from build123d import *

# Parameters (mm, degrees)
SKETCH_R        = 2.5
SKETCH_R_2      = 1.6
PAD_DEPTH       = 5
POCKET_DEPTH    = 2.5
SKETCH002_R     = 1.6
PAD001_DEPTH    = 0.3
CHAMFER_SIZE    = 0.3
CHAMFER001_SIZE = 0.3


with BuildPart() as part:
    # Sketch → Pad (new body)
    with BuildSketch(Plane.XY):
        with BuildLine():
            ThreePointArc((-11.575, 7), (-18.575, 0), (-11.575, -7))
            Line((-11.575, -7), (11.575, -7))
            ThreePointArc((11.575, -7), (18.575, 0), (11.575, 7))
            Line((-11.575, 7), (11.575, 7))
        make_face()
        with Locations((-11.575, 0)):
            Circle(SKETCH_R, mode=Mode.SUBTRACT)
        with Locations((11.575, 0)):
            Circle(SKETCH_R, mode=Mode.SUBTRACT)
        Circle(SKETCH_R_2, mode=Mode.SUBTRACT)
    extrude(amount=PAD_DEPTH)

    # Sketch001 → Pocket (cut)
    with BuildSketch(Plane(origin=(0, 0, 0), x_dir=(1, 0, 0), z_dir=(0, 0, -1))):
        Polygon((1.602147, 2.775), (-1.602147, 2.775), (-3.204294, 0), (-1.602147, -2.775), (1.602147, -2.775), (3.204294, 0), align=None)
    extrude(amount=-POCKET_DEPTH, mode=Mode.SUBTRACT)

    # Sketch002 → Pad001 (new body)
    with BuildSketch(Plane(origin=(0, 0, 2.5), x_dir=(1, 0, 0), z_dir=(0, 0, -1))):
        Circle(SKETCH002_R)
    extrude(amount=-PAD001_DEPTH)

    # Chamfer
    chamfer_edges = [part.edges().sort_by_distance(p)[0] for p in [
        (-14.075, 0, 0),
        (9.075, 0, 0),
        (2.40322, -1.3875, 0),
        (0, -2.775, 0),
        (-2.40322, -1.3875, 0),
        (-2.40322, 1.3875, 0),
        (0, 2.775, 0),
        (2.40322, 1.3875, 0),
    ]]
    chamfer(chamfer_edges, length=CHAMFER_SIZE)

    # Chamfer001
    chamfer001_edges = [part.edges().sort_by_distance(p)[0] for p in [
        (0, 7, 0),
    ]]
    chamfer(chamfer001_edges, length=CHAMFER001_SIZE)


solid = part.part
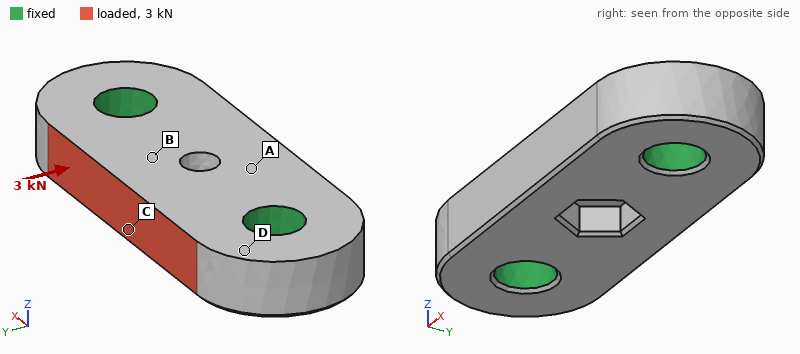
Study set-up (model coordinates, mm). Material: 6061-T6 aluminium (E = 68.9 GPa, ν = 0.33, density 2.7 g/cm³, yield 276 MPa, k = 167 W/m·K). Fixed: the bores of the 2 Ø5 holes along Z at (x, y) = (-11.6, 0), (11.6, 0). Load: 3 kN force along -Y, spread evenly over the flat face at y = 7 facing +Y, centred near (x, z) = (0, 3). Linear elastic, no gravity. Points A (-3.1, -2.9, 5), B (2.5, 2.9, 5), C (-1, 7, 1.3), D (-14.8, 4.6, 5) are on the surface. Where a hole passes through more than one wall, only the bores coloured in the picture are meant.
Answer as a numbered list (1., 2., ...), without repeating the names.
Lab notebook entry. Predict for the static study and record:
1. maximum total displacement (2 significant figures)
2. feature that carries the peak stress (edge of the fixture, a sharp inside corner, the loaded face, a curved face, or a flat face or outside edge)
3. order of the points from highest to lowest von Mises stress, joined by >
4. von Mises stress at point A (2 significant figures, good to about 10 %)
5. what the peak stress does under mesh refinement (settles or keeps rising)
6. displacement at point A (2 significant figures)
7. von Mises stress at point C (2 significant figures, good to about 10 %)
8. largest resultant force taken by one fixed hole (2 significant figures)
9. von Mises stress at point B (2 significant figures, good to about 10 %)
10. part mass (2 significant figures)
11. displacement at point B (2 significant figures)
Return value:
1. 8.6 µm
2. edge of the fixture
3. C > B > A > D
4. 17 MPa
5. keeps rising
6. 5.1 µm
7. 38 MPa
8. 1.5 kN
9. 26 MPa
10. 5.7 g
11. 6.8 µm
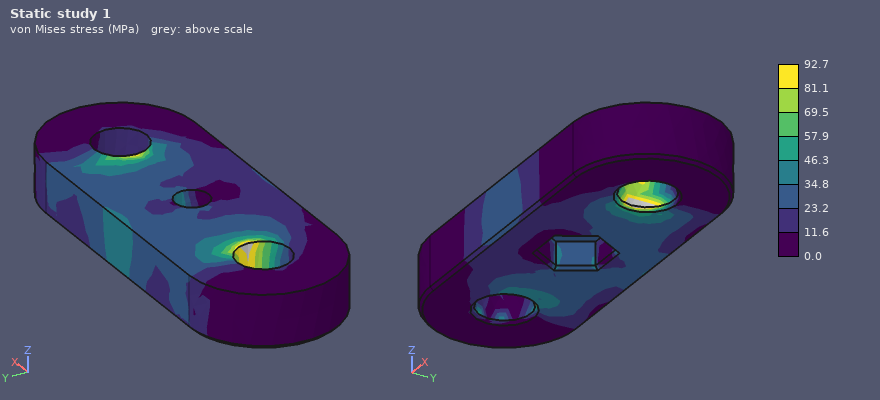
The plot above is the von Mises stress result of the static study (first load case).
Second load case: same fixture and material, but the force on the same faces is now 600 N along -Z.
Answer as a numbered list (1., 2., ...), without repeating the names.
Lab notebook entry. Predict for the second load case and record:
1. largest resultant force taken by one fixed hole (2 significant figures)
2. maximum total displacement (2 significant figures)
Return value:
1. 300 N
2. 11 µm
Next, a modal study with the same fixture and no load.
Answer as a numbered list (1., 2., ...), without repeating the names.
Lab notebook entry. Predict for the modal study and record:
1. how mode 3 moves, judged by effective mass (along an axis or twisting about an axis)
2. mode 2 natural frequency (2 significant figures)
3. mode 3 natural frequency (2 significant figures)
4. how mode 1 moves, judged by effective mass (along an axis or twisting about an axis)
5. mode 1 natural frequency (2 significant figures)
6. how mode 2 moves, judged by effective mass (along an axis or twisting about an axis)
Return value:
1. along Y
2. 47 kHz
3. 60 kHz
4. along Z
5. 44 kHz
6. twisting about X
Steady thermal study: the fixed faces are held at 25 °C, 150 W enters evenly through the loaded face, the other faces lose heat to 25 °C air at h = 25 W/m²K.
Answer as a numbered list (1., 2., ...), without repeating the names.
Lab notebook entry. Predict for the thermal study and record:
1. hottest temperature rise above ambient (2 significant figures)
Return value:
1. 74 K
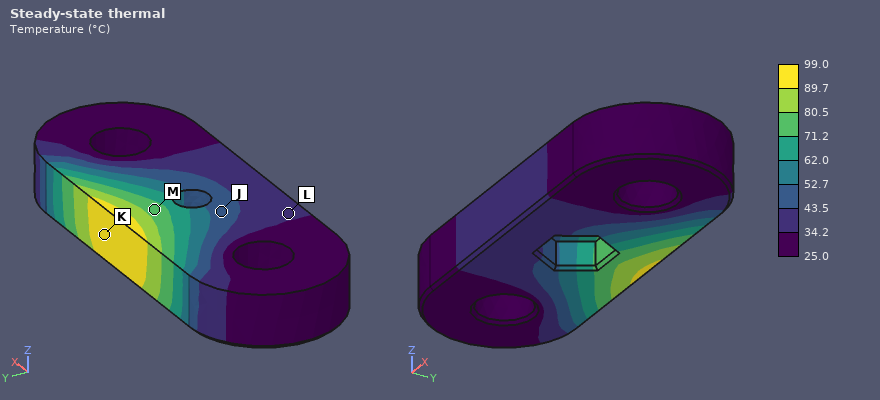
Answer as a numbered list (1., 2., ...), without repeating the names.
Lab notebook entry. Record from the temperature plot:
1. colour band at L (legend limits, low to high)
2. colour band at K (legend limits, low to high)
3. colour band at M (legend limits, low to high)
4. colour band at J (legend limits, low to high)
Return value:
1. 34.2 to 43.5 °C
2. 89.7 to 99.0 °C
3. 71.2 to 80.5 °C
4. 43.5 to 52.7 °C
